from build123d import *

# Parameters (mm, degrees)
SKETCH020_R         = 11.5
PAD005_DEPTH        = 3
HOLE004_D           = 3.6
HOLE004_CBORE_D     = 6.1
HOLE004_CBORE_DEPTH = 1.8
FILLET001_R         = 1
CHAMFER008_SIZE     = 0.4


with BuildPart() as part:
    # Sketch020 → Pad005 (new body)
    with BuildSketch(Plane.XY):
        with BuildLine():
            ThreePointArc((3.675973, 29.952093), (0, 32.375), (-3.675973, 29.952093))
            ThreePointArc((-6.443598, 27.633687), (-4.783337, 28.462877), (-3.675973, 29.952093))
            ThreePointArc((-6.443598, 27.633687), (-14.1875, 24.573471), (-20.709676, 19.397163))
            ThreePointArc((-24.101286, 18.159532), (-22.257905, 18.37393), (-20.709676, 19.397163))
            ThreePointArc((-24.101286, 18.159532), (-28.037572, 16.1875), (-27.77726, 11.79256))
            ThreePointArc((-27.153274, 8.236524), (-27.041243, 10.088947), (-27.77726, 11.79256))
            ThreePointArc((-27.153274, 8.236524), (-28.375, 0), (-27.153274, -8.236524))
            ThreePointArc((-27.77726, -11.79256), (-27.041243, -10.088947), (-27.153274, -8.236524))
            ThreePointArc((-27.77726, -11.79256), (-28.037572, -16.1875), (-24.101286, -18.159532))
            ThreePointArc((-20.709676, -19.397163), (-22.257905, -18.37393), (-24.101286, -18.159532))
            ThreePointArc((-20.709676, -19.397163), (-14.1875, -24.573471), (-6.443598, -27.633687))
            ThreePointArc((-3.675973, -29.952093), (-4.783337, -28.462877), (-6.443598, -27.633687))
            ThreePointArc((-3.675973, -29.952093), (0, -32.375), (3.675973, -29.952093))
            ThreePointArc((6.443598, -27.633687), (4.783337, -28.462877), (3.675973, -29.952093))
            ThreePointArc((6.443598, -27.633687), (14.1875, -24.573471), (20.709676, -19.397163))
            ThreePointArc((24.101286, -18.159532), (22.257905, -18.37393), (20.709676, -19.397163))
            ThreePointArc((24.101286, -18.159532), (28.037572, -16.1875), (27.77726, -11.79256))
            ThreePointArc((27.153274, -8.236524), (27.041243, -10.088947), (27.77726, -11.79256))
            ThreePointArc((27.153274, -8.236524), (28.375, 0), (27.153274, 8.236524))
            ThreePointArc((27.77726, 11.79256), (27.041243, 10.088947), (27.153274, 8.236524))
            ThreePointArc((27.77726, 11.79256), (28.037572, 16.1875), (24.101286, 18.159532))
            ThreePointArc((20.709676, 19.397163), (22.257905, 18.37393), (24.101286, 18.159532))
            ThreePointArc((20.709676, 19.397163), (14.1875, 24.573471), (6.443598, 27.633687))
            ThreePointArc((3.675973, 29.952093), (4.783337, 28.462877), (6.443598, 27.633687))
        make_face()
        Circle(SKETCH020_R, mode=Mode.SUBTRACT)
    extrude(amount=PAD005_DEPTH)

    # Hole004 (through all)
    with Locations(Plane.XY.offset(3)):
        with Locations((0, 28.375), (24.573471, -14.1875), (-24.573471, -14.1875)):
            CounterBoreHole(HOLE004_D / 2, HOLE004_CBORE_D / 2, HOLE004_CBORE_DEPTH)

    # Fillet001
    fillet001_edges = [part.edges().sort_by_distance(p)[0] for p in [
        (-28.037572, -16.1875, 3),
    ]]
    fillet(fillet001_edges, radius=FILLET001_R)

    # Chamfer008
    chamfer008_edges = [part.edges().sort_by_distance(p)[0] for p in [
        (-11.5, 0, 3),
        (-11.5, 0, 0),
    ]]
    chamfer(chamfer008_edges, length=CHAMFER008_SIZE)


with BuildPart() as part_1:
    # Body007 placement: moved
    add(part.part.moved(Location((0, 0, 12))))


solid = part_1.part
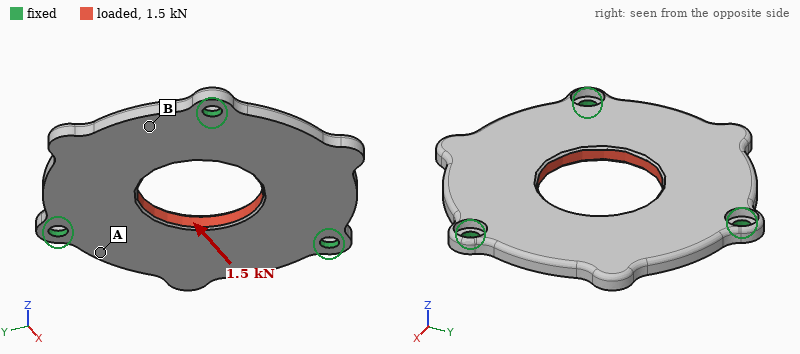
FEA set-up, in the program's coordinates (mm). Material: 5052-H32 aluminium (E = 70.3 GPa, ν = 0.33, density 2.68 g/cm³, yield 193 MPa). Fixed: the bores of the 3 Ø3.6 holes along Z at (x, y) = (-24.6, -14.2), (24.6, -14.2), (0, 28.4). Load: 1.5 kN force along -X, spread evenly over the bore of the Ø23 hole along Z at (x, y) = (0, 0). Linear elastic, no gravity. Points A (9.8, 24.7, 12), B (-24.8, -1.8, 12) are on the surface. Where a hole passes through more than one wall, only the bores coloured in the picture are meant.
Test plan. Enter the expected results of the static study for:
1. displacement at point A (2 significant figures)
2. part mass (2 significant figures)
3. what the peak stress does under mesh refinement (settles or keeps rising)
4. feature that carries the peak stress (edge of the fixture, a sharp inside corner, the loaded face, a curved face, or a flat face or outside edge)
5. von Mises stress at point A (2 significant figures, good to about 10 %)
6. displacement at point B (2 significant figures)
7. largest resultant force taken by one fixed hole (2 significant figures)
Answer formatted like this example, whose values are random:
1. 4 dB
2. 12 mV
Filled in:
1. 8.7 µm
2. 18 g
3. keeps rising
4. edge of the fixture
5. 19 MPa
6. 6.4 µm
7. 500 N
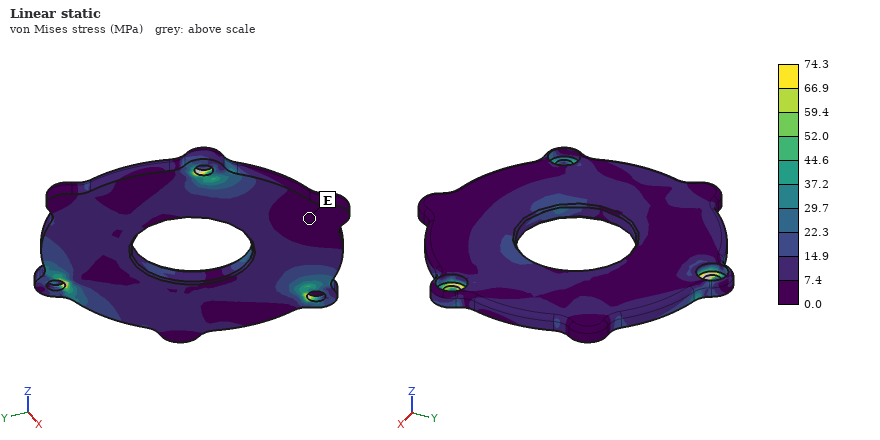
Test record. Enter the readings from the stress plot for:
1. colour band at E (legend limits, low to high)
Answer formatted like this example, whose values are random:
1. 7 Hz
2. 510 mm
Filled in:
1. 0.0 to 7.4 MPa
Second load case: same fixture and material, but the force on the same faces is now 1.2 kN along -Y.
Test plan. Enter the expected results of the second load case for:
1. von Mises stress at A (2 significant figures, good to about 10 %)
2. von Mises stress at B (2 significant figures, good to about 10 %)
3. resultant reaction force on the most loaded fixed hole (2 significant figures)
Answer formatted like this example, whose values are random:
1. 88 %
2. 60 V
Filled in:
1. 5.8 MPa
2. 13 MPa
3. 410 N
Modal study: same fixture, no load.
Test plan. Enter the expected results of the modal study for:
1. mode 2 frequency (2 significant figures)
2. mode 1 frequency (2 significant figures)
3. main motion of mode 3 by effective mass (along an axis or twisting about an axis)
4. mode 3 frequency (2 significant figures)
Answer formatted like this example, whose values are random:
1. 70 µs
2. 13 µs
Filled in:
1. 3800 Hz
2. 3800 Hz
3. along Z
4. 4600 Hz
